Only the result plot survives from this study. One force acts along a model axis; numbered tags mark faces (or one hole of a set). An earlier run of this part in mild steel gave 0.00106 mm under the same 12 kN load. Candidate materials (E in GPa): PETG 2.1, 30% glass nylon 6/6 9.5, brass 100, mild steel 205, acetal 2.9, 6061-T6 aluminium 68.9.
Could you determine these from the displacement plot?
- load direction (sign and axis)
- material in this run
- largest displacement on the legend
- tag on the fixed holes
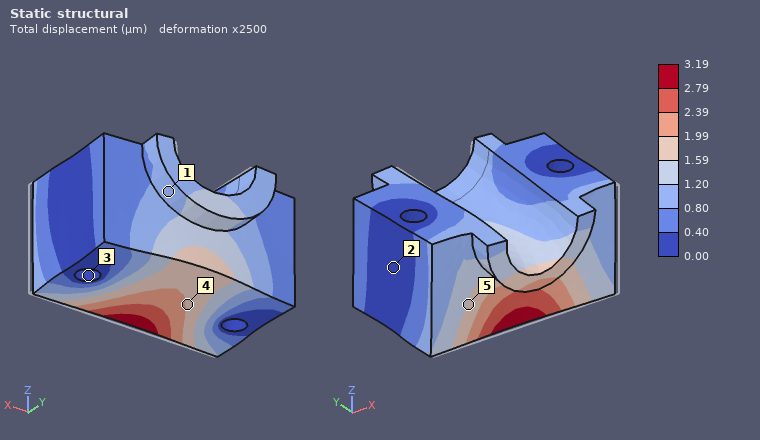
+Y
6061-T6 aluminium
3.19 µm
3
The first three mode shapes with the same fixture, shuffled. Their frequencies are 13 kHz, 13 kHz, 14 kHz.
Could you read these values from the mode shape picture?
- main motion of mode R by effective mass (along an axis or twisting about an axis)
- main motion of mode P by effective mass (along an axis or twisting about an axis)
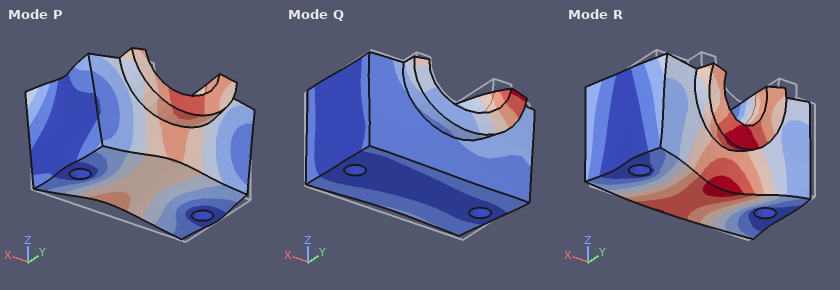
along Y
along Z
